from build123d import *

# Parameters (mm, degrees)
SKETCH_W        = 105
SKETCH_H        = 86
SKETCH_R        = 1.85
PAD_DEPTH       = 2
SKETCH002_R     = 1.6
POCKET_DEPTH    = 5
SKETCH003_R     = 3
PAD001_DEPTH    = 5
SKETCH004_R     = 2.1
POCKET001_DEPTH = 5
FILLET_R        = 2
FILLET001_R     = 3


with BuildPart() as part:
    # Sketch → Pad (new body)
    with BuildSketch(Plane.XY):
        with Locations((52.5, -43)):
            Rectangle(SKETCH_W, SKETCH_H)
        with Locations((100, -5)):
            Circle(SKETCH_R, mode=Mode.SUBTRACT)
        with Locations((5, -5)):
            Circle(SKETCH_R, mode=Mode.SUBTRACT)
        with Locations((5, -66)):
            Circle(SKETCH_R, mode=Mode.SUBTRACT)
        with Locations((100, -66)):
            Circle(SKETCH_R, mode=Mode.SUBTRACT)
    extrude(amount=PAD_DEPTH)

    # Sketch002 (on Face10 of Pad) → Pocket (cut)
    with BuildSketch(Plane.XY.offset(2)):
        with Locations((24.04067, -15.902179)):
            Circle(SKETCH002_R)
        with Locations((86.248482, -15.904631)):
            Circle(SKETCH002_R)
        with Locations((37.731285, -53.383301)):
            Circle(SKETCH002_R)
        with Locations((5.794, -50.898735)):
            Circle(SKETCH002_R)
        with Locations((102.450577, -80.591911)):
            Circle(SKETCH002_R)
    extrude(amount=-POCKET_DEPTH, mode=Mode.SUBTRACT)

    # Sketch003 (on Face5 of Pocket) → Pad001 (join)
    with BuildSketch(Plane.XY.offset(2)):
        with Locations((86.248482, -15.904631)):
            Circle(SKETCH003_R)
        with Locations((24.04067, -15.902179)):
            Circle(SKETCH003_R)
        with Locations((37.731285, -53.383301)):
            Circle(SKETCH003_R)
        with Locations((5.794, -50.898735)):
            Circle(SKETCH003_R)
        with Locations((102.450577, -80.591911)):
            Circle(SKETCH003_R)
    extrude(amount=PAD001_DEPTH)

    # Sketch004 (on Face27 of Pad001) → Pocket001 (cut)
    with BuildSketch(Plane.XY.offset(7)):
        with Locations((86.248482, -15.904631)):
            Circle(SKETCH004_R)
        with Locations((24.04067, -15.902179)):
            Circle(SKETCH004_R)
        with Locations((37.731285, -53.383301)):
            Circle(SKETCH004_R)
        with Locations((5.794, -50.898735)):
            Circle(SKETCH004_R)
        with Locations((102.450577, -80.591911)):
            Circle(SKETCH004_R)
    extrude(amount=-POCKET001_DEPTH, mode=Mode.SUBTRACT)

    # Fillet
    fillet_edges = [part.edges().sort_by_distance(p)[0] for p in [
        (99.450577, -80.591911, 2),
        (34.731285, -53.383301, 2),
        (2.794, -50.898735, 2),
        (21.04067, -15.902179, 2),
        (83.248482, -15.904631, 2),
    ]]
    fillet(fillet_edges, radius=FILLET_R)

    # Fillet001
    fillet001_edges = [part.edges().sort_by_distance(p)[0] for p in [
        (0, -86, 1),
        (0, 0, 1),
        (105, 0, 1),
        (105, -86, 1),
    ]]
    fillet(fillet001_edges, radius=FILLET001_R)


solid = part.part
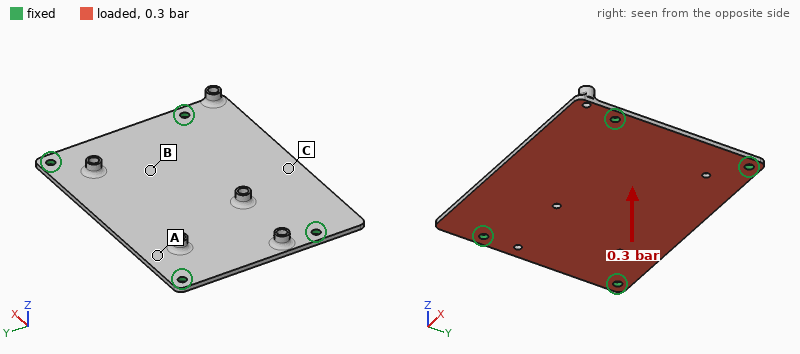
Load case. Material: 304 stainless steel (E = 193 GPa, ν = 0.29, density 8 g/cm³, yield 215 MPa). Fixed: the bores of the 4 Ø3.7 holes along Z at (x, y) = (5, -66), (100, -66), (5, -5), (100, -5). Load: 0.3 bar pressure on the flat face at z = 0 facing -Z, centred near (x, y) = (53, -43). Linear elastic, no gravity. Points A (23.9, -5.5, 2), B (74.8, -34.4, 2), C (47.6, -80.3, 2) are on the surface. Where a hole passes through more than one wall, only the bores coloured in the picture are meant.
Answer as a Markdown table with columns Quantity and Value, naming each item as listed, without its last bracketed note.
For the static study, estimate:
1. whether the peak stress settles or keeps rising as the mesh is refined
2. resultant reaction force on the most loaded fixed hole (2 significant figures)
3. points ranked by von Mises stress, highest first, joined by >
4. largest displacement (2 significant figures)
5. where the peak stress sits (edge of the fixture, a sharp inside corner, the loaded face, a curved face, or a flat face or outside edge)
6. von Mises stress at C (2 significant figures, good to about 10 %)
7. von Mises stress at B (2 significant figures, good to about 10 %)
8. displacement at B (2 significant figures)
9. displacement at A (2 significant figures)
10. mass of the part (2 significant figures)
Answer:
| Quantity | Value |
|---|---|
| whether the peak stress settles or keeps rising as the mesh is refined | keeps rising |
| resultant reaction force on the most loaded fixed hole | 81 N |
| points ranked by von Mises stress, highest first, joined by > | C > B > A |
| largest displacement | 72 µm |
| where the peak stress sits | edge of the fixture |
| von Mises stress at C | 20 MPa |
| von Mises stress at B | 10 MPa |
| displacement at B | 53 µm |
| displacement at A | 28 µm |
| mass of the part | 150 g |
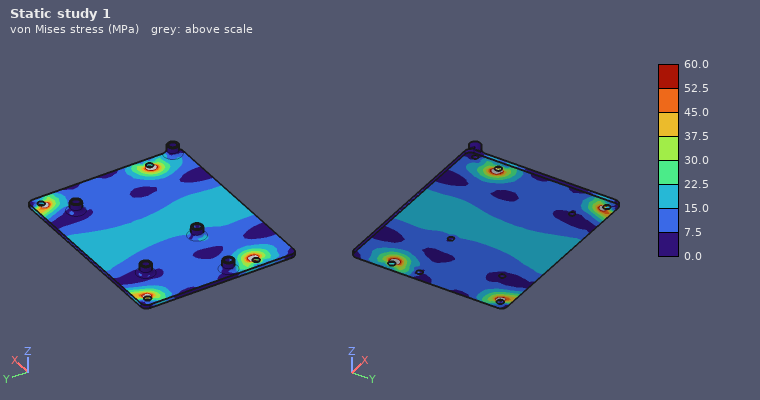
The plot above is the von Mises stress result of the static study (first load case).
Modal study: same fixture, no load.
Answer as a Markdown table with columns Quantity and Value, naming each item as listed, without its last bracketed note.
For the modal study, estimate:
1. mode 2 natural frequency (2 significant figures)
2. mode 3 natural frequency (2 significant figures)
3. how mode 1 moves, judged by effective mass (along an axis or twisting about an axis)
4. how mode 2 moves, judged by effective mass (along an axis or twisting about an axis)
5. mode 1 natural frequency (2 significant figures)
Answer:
| Quantity | Value |
|---|---|
| mode 2 natural frequency | 1300 Hz |
| mode 3 natural frequency | 2100 Hz |
| how mode 1 moves, judged by effective mass | along Z |
| how mode 2 moves, judged by effective mass | twisting about X |
| mode 1 natural frequency | 930 Hz |
